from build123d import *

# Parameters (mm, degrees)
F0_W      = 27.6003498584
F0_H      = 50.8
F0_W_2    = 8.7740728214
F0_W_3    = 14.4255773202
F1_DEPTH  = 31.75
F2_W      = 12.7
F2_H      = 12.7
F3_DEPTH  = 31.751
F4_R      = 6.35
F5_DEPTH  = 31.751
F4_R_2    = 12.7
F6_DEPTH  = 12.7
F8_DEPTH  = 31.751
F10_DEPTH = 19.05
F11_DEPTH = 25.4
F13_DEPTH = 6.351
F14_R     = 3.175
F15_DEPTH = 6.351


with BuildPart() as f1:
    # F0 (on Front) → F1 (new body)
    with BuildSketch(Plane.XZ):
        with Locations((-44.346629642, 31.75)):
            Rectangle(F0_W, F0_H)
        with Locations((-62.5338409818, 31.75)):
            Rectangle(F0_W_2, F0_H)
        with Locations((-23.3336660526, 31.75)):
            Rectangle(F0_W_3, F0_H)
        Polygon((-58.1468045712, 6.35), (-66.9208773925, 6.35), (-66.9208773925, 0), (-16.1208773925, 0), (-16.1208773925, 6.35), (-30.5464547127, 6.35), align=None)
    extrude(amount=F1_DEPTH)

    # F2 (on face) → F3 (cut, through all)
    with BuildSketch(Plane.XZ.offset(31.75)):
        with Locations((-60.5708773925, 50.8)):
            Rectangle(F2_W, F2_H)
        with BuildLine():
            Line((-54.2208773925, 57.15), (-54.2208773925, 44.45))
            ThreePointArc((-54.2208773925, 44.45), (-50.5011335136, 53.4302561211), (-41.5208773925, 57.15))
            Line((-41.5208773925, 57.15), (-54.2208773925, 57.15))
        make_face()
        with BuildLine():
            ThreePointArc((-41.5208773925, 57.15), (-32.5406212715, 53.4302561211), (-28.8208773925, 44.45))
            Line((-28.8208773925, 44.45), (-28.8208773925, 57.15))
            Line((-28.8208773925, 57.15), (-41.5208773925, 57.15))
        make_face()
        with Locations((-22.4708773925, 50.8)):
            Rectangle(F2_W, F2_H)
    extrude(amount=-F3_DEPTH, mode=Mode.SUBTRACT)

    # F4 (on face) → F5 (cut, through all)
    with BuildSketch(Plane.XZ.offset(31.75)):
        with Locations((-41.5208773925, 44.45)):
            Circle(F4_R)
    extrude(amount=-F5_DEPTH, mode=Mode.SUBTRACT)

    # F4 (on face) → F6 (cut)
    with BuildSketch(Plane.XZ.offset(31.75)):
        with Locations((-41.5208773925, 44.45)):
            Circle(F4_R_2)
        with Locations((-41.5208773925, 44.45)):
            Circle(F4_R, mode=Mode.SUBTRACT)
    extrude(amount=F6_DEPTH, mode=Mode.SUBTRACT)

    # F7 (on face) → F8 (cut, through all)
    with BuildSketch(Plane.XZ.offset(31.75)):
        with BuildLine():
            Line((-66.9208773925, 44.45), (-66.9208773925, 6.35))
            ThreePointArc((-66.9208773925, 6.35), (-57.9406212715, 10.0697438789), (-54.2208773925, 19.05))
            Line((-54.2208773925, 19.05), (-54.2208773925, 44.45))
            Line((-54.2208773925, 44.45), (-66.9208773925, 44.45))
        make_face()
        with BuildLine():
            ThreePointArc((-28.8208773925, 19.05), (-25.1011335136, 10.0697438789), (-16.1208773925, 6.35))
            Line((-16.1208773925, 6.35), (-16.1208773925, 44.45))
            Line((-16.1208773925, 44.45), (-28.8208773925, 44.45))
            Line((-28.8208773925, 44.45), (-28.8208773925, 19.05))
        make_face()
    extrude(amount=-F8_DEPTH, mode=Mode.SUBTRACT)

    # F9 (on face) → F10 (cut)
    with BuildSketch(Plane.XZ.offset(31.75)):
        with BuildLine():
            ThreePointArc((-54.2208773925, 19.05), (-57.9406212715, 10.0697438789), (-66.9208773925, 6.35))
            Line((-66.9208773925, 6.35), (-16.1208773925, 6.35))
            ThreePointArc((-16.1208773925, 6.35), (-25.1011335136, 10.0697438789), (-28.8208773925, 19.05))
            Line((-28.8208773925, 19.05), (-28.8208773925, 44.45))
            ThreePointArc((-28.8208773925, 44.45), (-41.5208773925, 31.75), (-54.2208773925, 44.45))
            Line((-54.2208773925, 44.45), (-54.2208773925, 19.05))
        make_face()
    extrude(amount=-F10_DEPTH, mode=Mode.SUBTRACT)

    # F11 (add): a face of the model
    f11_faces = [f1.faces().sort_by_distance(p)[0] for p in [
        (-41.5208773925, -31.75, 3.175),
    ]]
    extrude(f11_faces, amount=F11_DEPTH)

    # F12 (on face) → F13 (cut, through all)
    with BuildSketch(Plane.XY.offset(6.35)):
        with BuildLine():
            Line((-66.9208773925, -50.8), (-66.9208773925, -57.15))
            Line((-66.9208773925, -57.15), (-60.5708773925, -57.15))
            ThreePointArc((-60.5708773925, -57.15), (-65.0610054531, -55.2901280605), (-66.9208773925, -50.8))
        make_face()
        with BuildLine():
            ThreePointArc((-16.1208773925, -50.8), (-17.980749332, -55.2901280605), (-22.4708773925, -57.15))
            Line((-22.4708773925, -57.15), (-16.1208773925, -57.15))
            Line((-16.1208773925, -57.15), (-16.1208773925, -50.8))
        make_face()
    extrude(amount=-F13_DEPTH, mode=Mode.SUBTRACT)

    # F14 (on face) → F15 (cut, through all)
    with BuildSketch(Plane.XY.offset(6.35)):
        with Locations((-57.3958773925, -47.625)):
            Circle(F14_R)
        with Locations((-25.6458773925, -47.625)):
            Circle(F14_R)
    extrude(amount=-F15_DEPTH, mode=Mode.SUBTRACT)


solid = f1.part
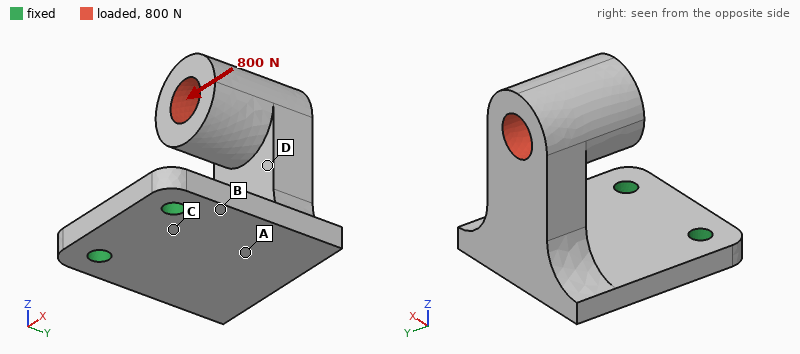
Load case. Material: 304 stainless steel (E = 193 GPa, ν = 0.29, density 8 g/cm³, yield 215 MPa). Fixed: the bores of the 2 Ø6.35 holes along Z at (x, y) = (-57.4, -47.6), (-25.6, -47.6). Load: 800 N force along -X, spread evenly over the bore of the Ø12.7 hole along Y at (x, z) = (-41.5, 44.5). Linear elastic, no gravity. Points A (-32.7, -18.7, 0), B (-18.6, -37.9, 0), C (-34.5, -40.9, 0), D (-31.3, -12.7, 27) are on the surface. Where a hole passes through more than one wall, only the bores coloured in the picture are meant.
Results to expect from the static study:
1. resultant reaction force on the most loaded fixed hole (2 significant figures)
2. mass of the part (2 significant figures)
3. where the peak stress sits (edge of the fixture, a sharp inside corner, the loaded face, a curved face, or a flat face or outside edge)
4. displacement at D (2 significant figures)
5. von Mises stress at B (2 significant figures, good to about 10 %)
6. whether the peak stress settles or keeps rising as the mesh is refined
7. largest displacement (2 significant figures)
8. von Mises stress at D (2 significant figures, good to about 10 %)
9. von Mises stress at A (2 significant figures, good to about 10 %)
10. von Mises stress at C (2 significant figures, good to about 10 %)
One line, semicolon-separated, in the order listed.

1.2 kN; 320 g; edge of the fixture; 0.060 mm; 56 MPa; keeps rising; 0.13 mm; 15 MPa; 47 MPa; 32 MPa
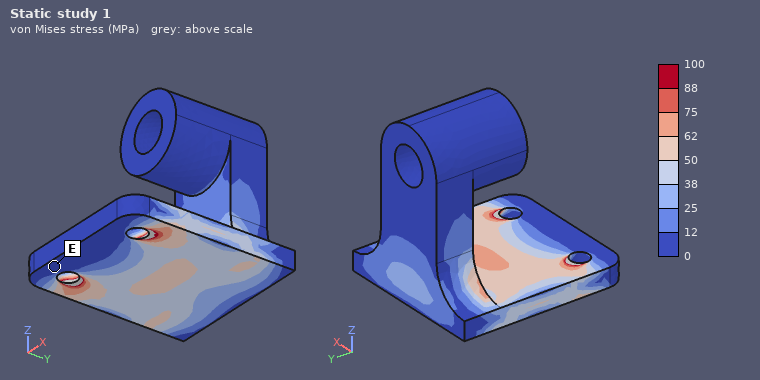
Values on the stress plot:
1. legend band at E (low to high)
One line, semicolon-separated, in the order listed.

0 to 12 MPa
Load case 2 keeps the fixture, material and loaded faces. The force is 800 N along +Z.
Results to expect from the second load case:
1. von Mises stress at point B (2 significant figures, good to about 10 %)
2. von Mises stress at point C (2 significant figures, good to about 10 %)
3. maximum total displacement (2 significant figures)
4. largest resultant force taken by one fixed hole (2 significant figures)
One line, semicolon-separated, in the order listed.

54 MPa; 44 MPa; 0.11 mm; 400 N
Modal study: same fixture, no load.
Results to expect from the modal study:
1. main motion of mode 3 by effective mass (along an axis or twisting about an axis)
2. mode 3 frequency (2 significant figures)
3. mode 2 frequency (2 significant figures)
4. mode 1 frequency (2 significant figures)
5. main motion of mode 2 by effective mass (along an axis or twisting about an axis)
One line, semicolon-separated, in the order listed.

along Z; 2200 Hz; 1300 Hz; 700 Hz; along X
